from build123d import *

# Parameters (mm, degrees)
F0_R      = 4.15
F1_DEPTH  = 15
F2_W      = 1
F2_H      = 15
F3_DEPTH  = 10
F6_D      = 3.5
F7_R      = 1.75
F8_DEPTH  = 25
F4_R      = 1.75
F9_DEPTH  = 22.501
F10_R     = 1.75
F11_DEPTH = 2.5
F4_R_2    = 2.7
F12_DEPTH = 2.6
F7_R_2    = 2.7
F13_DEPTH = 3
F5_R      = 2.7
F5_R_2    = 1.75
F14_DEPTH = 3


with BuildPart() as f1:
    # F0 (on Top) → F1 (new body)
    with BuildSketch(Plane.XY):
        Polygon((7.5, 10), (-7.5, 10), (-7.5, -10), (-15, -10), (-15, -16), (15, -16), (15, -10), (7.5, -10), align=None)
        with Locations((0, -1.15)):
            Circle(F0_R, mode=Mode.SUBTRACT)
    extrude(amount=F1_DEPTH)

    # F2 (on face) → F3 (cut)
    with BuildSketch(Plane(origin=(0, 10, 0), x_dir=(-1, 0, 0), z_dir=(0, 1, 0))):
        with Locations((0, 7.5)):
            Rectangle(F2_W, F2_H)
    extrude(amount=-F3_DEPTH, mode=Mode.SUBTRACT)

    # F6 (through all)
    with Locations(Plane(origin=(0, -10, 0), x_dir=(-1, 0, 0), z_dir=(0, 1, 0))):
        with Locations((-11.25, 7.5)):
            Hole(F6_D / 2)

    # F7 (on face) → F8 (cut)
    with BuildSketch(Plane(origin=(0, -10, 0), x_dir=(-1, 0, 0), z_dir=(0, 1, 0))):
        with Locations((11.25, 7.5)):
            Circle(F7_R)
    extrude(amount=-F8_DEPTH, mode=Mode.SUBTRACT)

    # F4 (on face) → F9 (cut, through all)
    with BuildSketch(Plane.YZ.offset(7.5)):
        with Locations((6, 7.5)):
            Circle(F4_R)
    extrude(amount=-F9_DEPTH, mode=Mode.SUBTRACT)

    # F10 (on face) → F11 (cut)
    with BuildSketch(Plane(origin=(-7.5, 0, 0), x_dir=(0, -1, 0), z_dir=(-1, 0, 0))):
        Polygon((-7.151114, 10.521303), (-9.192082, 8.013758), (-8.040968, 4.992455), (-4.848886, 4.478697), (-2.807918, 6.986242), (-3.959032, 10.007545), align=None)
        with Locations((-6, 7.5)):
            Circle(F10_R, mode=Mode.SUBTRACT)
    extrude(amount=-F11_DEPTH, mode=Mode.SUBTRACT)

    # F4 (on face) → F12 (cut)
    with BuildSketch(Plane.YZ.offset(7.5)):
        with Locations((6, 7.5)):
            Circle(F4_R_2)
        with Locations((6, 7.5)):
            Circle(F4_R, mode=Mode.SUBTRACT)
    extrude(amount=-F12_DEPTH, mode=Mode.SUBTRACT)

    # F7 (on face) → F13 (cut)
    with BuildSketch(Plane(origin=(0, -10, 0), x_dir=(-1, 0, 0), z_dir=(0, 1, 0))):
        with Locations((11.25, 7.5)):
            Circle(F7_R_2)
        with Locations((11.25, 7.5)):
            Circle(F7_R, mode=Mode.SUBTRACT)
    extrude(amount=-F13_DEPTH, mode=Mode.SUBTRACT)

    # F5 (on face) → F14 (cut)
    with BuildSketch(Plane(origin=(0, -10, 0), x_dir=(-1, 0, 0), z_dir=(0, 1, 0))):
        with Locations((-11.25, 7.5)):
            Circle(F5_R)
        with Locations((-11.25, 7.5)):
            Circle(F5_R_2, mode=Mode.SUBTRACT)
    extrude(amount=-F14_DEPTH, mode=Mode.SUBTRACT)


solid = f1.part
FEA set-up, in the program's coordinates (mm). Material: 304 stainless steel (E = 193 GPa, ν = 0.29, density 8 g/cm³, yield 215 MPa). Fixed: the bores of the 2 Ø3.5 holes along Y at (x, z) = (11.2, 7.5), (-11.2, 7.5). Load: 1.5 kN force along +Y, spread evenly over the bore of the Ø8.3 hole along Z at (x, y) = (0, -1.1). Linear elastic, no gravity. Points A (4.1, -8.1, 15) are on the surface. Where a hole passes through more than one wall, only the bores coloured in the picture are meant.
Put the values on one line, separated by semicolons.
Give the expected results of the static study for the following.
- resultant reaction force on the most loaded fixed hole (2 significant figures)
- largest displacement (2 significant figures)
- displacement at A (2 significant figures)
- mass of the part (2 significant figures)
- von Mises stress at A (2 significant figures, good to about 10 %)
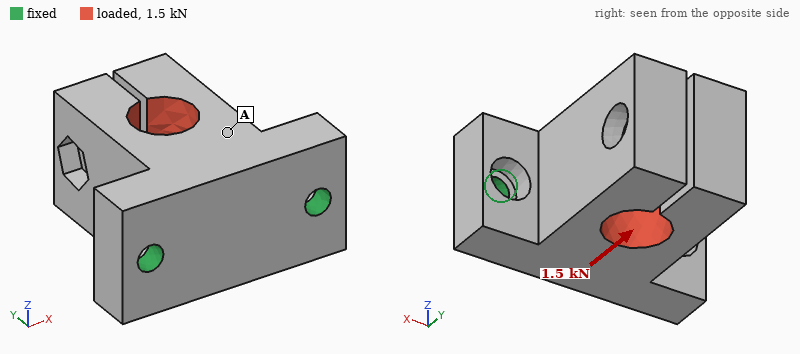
860 N; 11 µm; 1.9 µm; 47 g; 15 MPa
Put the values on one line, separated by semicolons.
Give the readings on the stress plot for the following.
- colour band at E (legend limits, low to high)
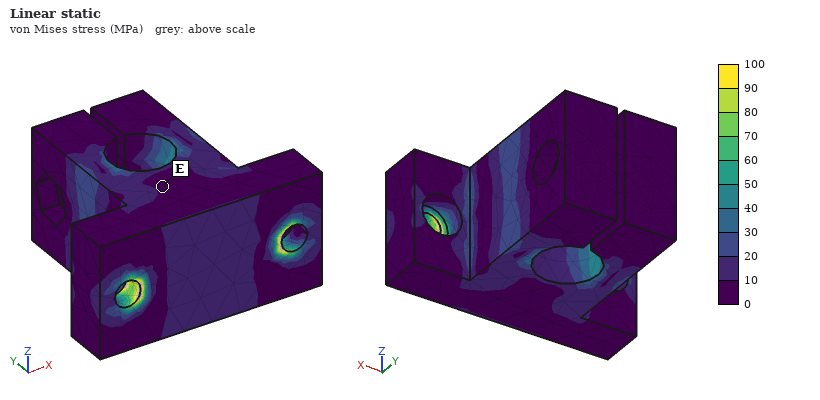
0 to 10 MPa
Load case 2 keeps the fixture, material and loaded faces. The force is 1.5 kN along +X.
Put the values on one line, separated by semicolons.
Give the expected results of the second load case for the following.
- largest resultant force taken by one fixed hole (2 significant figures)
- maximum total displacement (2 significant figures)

1.2 kN; 19 µm
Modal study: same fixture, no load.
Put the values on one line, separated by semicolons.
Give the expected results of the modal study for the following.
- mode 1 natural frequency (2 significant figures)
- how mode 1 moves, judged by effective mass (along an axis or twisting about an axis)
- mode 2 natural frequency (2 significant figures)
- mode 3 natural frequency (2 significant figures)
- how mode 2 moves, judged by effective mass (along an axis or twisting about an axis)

5400 Hz; along Z; 8000 Hz; 8500 Hz; along X
